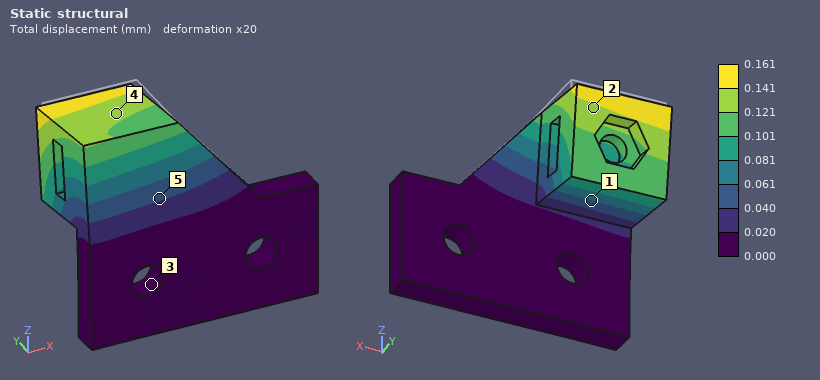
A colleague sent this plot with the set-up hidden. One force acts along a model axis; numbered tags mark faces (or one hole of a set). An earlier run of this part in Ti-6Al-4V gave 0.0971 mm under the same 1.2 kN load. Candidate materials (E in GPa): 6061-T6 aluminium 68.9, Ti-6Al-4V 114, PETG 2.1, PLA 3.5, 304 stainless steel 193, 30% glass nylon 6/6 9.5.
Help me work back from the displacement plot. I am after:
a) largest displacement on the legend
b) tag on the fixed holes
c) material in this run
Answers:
0.161 mm
3
6061-T6 aluminium
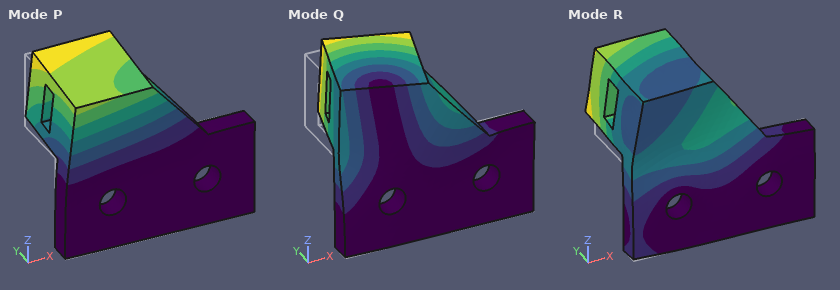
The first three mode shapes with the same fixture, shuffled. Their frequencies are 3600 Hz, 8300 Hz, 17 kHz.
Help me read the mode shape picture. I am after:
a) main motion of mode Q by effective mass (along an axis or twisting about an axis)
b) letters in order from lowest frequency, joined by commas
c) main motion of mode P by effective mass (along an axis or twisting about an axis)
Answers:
along X
P, Q, R
along Y
